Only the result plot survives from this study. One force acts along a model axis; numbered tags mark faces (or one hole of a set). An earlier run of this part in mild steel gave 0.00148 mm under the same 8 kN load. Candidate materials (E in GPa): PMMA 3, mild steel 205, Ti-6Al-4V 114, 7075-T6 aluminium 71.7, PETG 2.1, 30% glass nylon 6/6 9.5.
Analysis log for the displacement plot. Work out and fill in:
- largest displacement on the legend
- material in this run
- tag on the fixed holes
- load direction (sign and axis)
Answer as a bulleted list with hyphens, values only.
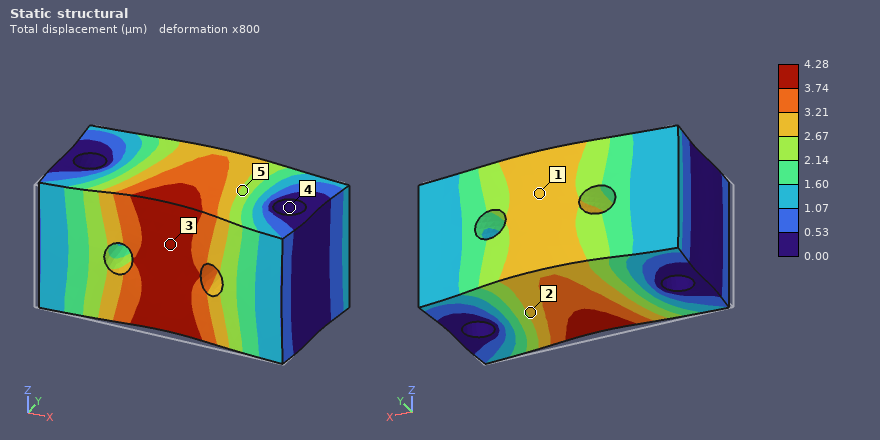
- 4.28 µm
- 7075-T6 aluminium
- 4
- +Y
